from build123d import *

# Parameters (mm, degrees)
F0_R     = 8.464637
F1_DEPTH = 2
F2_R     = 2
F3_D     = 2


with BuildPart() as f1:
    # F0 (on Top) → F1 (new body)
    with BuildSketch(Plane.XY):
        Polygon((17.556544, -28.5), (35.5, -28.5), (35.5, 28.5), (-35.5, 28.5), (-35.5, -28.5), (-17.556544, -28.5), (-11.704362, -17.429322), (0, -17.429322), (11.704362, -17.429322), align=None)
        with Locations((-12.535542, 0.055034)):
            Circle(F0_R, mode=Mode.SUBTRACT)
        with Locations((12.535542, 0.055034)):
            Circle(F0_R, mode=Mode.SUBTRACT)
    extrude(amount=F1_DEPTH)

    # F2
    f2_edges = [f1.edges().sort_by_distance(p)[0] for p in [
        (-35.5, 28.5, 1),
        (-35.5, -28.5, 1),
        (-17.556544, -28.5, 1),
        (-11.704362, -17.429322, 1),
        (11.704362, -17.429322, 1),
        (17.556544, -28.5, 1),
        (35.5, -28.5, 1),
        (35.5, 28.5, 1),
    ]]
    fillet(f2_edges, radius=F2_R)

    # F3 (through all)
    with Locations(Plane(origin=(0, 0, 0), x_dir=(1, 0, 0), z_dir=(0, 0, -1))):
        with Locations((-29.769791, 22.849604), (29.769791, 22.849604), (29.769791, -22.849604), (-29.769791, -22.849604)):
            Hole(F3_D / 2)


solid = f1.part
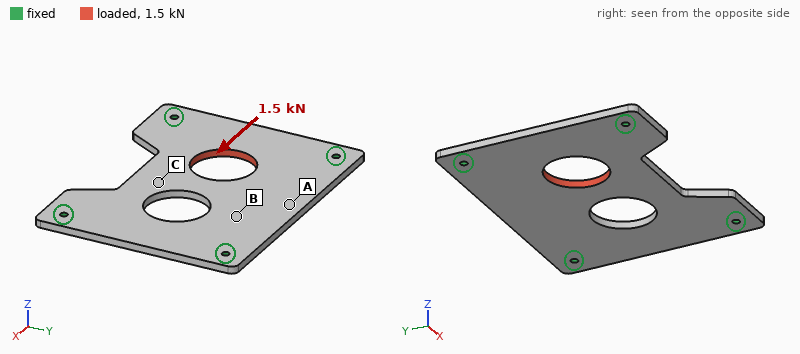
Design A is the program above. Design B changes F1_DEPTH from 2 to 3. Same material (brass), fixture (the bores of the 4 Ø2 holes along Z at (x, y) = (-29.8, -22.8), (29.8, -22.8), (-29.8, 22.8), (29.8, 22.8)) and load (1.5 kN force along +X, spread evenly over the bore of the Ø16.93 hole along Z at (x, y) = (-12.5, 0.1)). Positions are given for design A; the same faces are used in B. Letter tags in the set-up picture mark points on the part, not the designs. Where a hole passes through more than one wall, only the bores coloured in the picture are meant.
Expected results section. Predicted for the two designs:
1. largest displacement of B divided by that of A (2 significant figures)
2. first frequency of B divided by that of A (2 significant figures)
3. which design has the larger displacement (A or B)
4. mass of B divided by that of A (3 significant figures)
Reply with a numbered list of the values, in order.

1. 0.66
2. 1.4
3. A
4. 1.50
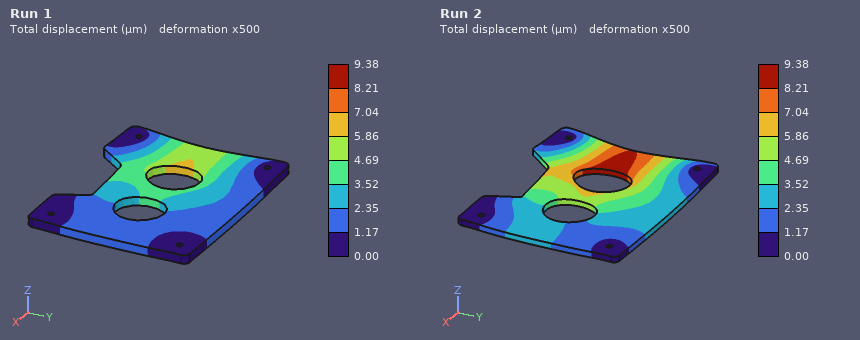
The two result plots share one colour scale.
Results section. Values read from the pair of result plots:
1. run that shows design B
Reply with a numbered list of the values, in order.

1. Run 1
